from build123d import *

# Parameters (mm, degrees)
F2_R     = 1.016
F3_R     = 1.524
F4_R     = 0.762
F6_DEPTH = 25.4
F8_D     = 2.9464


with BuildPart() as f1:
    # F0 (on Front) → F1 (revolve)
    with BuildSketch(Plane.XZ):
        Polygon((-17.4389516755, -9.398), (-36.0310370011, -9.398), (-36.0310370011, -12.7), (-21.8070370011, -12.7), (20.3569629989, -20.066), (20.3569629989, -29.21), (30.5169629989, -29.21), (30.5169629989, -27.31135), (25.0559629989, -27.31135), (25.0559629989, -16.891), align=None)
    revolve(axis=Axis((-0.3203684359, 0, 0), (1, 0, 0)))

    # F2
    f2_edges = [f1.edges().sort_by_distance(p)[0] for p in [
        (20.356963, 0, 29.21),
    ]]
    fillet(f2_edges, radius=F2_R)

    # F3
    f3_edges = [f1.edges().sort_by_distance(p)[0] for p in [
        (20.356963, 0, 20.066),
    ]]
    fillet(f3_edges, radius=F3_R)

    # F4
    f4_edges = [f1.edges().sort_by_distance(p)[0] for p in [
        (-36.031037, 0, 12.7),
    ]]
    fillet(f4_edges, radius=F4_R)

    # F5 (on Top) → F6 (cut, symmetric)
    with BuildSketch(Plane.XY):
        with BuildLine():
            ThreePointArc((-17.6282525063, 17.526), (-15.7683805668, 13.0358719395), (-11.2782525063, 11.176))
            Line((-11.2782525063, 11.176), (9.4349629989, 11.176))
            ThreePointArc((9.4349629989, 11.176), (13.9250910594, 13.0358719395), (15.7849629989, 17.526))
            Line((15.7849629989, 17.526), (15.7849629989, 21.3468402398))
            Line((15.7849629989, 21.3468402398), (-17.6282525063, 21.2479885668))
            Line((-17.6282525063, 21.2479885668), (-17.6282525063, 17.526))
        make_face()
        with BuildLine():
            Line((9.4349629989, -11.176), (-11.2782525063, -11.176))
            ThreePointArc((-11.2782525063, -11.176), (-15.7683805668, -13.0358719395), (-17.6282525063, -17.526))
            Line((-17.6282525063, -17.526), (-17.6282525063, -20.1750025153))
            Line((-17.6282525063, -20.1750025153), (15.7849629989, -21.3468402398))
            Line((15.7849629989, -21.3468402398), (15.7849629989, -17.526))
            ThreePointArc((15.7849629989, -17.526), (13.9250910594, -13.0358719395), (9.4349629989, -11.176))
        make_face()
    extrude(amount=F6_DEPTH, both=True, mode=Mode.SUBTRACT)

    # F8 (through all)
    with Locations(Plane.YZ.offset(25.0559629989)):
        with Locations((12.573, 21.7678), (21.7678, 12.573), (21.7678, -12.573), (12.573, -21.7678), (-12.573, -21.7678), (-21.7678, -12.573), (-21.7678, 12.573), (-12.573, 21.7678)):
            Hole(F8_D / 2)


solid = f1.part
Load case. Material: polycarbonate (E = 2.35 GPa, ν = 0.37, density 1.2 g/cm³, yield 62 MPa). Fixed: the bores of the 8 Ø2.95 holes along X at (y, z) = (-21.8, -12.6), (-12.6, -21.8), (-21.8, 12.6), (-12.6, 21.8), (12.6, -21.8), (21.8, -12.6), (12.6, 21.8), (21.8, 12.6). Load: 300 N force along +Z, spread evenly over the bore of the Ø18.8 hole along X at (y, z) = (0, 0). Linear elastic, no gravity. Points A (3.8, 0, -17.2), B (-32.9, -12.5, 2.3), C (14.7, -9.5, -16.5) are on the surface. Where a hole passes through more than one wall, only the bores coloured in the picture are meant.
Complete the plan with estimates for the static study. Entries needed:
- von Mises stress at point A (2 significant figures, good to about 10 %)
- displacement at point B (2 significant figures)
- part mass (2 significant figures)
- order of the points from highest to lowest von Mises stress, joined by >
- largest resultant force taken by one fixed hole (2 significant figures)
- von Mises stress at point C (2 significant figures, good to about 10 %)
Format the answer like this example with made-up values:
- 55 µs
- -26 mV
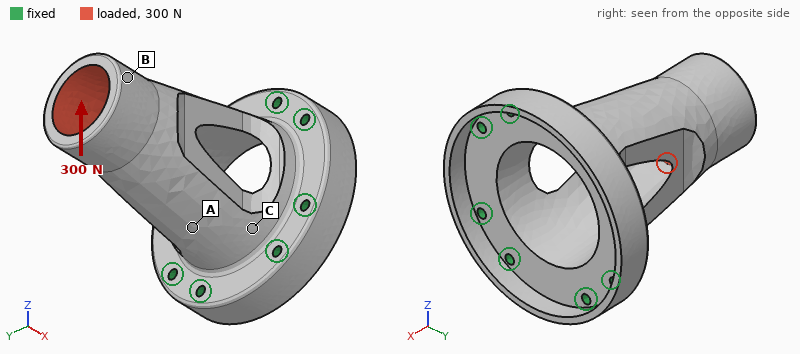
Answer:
- 3.4 MPa
- 0.47 mm
- 29 g
- C > A > B
- 190 N
- 9.2 MPa
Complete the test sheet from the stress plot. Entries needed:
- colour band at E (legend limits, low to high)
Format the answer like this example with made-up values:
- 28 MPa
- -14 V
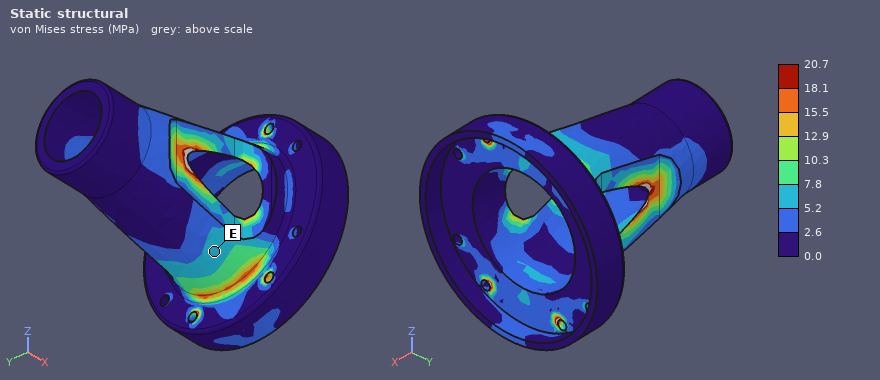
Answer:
- 5.2 to 7.8 MPa
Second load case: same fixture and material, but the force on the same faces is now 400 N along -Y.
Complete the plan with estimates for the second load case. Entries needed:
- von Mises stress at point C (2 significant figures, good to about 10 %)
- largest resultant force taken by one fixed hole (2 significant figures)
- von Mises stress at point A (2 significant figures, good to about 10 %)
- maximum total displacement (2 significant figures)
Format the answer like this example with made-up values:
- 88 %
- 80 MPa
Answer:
- 11 MPa
- 200 N
- 5.0 MPa
- 1.1 mm
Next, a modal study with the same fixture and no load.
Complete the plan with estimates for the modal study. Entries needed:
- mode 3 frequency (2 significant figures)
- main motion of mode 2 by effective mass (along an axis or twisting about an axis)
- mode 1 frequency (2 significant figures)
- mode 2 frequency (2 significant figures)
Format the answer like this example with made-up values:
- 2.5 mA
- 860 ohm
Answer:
- 3000 Hz
- along Z
- 1300 Hz
- 1400 Hz
